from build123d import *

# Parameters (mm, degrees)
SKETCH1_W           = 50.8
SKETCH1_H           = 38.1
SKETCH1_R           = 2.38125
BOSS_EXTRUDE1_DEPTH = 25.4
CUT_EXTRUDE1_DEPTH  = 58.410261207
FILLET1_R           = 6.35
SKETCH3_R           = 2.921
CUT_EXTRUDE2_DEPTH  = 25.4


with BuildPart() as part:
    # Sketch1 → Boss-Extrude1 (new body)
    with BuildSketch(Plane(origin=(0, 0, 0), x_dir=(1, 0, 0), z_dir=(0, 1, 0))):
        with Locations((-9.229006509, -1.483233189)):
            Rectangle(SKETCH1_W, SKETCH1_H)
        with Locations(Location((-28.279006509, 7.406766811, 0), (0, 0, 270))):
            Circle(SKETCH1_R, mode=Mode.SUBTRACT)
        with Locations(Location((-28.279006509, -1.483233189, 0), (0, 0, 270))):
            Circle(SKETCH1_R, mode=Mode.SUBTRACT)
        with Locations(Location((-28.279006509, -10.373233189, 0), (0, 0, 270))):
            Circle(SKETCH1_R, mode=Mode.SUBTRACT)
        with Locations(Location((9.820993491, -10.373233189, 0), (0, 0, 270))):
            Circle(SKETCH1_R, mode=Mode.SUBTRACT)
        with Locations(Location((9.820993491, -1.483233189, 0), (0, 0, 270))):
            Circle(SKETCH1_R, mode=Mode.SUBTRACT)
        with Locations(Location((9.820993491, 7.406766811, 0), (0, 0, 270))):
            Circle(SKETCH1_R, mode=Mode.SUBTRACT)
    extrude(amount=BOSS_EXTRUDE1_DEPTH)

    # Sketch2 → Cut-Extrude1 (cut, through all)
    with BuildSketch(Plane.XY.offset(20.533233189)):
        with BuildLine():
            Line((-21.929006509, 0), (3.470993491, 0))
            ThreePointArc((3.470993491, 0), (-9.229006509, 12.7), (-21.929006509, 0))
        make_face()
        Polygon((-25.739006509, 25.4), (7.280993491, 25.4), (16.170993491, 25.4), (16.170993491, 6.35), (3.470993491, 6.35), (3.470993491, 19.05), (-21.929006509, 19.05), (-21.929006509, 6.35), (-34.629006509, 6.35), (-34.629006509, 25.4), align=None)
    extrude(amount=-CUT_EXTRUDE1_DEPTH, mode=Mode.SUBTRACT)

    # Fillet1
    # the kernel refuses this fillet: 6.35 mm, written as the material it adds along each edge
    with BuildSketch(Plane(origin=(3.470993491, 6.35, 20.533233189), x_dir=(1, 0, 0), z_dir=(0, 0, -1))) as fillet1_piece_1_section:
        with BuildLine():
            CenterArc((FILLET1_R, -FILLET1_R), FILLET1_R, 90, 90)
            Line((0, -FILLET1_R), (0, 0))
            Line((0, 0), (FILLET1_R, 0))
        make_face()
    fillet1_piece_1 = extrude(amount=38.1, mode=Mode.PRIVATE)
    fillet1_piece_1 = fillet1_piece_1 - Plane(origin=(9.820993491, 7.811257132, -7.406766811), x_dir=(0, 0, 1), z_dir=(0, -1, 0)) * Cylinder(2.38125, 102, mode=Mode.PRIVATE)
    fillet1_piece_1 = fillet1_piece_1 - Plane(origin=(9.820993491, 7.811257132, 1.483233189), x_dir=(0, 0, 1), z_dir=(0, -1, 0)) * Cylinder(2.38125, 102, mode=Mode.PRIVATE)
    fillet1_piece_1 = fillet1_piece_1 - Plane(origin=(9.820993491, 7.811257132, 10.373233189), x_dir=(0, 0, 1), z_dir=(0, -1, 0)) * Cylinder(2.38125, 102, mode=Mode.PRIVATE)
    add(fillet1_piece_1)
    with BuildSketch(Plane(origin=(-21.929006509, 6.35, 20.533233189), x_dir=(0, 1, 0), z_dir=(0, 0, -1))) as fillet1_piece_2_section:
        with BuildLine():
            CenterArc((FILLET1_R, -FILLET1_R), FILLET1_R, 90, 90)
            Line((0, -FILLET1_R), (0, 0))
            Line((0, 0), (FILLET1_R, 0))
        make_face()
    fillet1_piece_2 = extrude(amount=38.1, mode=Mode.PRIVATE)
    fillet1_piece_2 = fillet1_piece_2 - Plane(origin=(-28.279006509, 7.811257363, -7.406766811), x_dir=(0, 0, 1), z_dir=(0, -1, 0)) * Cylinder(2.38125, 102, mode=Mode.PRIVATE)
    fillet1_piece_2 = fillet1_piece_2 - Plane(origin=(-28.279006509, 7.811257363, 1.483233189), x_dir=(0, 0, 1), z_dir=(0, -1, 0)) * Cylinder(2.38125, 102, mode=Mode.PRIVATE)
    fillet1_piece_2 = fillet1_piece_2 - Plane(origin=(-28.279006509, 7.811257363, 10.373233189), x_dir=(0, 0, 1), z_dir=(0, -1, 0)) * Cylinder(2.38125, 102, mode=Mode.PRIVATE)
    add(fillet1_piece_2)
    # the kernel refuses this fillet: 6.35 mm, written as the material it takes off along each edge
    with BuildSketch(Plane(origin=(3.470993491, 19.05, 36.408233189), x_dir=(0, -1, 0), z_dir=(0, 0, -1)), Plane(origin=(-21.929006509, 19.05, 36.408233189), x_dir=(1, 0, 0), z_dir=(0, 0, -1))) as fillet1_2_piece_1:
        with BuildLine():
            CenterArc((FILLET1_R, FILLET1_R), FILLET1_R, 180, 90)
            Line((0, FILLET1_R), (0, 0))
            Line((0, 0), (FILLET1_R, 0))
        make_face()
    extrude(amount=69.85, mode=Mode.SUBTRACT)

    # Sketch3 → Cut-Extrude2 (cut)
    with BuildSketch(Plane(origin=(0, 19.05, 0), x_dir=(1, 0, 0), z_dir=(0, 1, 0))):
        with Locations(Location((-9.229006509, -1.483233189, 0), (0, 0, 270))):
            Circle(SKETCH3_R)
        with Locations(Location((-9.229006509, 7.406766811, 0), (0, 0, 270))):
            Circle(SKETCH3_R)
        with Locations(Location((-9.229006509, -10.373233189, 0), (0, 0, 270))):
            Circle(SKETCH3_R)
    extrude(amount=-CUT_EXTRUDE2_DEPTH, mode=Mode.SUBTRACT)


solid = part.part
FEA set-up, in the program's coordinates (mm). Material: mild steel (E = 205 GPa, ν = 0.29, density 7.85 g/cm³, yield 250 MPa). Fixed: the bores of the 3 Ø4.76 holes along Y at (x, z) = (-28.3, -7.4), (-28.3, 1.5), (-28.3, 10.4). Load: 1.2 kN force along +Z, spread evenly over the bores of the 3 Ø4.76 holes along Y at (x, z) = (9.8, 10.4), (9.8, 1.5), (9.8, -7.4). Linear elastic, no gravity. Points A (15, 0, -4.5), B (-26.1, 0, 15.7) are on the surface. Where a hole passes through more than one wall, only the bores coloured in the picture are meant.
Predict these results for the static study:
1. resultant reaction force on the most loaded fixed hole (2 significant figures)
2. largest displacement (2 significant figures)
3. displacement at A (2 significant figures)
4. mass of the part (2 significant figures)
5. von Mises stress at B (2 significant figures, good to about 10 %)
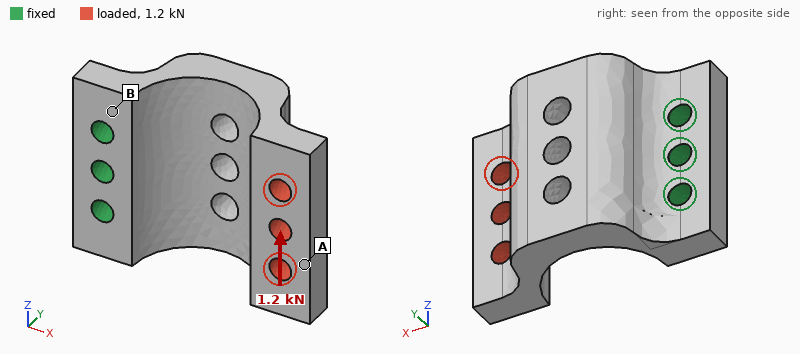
2.0 kN
88 µm
75 µm
110 g
38 MPa
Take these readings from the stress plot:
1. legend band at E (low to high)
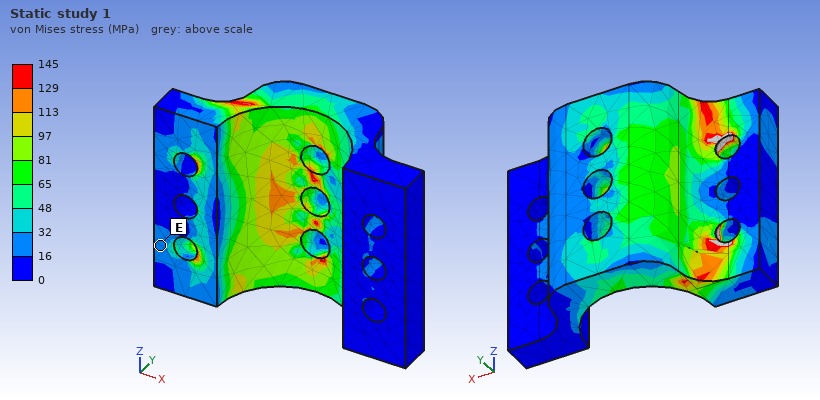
16 to 32 MPa
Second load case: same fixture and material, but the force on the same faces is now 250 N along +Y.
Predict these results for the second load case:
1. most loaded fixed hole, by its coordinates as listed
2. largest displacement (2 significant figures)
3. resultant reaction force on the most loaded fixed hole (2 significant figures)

(-28.3, 1.5)
78 µm
130 N
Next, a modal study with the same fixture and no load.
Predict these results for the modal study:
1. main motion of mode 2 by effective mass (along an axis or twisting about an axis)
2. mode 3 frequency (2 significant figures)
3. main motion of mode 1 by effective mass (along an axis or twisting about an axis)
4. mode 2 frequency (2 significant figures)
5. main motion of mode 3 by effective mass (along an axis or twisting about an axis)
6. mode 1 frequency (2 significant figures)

along Z
6100 Hz
along Y
3500 Hz
along X
1700 Hz
